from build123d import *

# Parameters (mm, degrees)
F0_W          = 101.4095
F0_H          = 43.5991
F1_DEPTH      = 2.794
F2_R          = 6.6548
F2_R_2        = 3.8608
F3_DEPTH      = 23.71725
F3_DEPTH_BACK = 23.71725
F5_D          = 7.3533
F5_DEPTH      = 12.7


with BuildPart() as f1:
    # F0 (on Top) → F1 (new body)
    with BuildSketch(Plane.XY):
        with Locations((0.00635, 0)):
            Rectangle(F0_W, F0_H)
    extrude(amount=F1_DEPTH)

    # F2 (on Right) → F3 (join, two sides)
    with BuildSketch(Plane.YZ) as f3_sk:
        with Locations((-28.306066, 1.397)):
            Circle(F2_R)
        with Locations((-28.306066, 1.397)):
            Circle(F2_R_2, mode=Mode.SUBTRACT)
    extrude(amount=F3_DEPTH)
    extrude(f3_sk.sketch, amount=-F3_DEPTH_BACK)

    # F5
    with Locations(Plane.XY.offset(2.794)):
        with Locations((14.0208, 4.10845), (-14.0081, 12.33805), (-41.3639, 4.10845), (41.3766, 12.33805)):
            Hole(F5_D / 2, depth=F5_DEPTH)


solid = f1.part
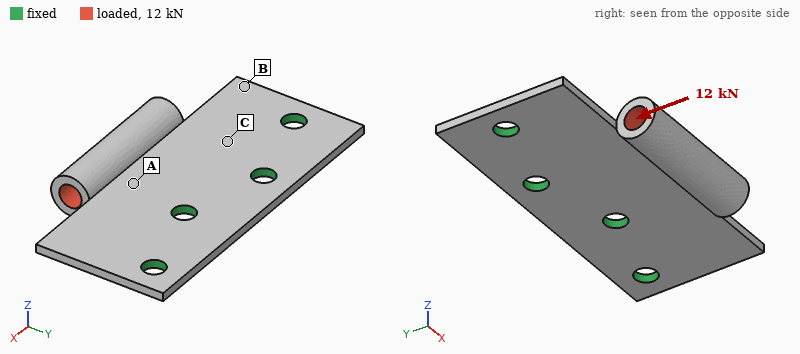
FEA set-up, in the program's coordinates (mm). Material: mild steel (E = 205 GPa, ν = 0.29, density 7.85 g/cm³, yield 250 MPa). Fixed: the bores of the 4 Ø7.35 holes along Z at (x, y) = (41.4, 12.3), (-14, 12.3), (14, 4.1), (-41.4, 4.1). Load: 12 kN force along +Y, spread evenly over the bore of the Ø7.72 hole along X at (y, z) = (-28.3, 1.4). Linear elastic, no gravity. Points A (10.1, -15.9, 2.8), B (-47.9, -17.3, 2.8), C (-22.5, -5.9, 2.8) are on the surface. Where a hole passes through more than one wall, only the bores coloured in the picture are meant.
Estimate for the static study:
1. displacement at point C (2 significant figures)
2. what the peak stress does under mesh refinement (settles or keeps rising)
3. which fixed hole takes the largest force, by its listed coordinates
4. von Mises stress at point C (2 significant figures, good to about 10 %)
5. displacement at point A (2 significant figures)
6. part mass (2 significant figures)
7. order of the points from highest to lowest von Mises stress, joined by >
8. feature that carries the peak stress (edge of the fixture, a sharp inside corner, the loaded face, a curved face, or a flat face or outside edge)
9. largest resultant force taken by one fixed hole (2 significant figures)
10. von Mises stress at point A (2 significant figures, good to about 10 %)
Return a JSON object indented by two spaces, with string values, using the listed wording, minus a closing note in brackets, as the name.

{
  "displacement at point C": "4.8 µm",
  "what the peak stress does under mesh refinement": "keeps rising",
  "which fixed hole takes the largest force, by its listed coordinates": "(14, 4.1)",
  "von Mises stress at point C": "53 MPa",
  "displacement at point A": "8.6 µm",
  "part mass": "130 g",
  "order of the points from highest to lowest von Mises stress, joined by >": "A > C > B",
  "feature that carries the peak stress": "a sharp inside corner",
  "largest resultant force taken by one fixed hole": "5.4 kN",
  "von Mises stress at point A": "84 MPa"
}
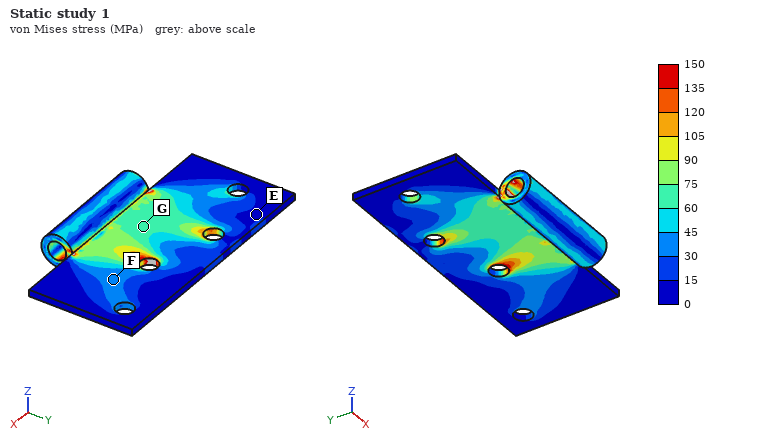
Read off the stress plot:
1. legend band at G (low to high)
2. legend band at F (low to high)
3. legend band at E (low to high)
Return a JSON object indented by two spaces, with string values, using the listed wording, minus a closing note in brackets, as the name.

{
  "legend band at G": "60 to 75 MPa",
  "legend band at F": "30 to 45 MPa",
  "legend band at E": "0 to 15 MPa"
}
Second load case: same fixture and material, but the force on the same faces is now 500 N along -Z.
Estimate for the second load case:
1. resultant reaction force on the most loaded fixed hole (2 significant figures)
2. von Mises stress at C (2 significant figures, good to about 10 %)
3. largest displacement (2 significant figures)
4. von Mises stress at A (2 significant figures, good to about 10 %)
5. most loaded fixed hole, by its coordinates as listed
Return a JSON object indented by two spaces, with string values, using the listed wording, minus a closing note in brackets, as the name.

{
  "resultant reaction force on the most loaded fixed hole": "390 N",
  "von Mises stress at C": "79 MPa",
  "largest displacement": "0.24 mm",
  "von Mises stress at A": "58 MPa",
  "most loaded fixed hole, by its coordinates as listed": "(14, 4.1)"
}
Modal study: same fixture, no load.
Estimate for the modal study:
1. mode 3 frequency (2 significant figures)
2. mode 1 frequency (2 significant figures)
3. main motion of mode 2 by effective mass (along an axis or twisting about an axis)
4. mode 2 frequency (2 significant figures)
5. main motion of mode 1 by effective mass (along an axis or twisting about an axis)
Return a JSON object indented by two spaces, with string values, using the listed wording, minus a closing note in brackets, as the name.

{
  "mode 3 frequency": "5000 Hz",
  "mode 1 frequency": "1300 Hz",
  "main motion of mode 2 by effective mass": "twisting about Y",
  "mode 2 frequency": "3100 Hz",
  "main motion of mode 1 by effective mass": "along Z"
}
